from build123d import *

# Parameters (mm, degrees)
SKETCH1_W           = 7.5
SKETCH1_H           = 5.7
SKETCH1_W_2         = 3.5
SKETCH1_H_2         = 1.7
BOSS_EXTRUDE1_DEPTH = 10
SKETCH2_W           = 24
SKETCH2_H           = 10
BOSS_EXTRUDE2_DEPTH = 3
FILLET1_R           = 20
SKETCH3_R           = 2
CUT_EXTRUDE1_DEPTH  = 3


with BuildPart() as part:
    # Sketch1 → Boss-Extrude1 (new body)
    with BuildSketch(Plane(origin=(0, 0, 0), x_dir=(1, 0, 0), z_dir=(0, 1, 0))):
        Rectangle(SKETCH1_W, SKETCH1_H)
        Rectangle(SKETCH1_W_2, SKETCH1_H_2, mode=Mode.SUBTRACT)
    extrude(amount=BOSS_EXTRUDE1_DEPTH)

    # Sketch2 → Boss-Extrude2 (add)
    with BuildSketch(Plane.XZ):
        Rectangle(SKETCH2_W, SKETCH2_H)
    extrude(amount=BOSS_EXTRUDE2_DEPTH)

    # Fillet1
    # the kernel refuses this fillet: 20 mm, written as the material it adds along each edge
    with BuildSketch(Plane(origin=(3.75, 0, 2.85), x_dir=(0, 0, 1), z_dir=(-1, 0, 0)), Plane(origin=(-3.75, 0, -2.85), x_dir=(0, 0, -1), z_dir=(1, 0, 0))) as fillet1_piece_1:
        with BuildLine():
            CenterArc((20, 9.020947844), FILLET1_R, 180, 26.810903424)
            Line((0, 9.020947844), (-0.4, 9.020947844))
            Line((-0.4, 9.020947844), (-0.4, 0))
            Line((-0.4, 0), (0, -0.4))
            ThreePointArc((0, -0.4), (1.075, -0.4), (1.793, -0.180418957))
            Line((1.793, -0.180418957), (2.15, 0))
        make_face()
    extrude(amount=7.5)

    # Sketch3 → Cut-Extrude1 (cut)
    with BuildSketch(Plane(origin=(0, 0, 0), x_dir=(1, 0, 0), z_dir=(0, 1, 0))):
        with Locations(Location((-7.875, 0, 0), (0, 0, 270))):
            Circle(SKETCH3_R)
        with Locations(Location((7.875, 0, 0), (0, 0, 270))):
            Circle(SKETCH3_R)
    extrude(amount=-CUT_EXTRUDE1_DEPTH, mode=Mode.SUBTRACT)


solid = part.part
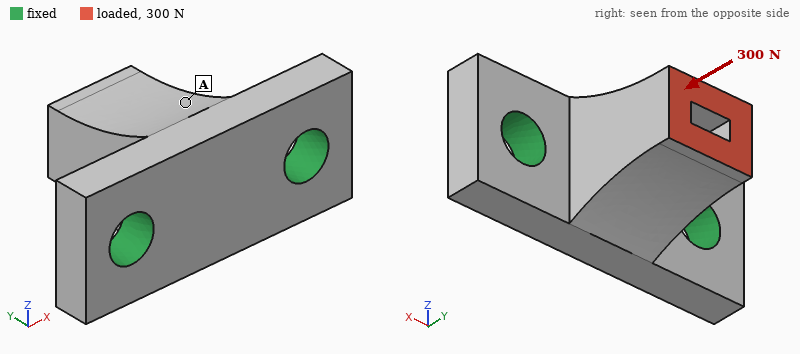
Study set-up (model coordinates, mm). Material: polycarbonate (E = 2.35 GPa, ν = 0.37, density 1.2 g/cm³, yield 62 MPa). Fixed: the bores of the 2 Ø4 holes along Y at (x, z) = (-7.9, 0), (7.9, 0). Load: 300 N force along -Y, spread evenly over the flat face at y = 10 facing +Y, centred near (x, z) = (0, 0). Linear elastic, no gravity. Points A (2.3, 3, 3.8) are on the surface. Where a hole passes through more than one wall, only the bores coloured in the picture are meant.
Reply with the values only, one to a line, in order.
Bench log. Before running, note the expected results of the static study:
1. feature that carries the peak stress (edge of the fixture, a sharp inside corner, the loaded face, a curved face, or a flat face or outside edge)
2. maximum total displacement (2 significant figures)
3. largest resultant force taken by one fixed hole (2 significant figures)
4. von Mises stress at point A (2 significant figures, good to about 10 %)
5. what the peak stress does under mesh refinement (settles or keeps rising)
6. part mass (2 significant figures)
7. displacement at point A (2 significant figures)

edge of the fixture
77 µm
160 N
5.3 MPa
keeps rising
1.3 g
52 µm
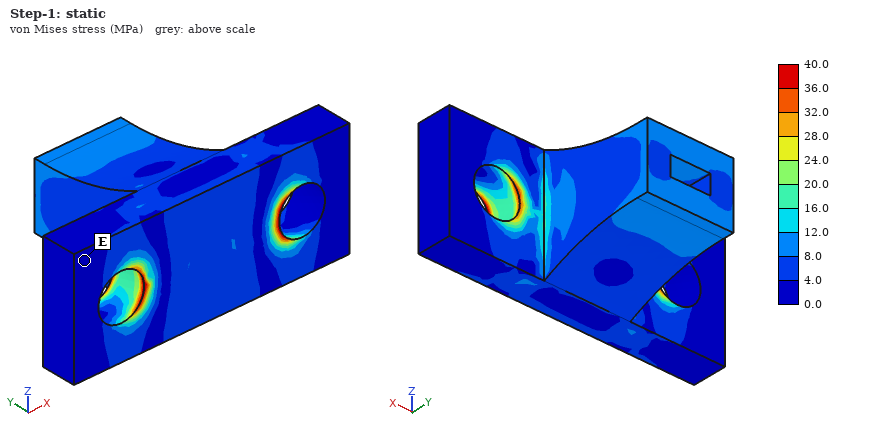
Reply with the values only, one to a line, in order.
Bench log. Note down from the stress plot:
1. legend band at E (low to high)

0.0 to 4.0 MPa
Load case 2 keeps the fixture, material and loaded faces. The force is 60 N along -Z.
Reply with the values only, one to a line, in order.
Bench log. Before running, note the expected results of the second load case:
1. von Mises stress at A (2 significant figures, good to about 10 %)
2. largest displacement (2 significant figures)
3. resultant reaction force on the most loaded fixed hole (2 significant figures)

7.4 MPa
0.23 mm
30 N
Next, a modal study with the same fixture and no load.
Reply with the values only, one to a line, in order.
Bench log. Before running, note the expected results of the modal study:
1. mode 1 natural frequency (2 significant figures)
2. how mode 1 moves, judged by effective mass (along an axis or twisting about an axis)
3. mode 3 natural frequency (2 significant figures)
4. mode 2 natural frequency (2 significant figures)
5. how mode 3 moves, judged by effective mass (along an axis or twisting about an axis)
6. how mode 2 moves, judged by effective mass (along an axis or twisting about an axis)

5900 Hz
along Z
13 kHz
9700 Hz
along Y
along X
